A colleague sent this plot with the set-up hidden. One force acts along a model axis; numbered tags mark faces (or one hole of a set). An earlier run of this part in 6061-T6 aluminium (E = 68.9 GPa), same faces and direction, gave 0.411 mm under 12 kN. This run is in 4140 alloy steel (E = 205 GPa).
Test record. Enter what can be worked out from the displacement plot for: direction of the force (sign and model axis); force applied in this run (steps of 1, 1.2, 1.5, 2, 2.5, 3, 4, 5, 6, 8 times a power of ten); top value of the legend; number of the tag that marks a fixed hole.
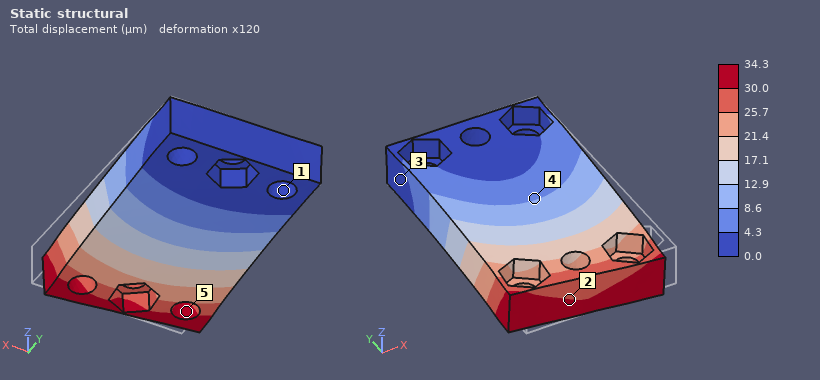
-X
3 kN
34.3 µm
1
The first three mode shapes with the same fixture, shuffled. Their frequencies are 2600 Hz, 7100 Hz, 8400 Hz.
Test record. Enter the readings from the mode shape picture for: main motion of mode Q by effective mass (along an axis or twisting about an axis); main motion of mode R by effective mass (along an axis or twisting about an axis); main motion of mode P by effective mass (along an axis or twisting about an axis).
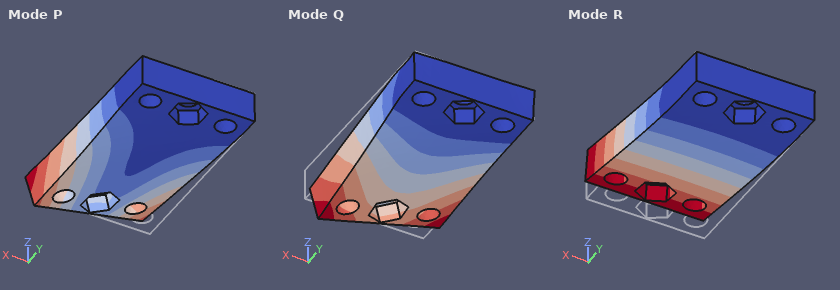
along X
along Z
along X
